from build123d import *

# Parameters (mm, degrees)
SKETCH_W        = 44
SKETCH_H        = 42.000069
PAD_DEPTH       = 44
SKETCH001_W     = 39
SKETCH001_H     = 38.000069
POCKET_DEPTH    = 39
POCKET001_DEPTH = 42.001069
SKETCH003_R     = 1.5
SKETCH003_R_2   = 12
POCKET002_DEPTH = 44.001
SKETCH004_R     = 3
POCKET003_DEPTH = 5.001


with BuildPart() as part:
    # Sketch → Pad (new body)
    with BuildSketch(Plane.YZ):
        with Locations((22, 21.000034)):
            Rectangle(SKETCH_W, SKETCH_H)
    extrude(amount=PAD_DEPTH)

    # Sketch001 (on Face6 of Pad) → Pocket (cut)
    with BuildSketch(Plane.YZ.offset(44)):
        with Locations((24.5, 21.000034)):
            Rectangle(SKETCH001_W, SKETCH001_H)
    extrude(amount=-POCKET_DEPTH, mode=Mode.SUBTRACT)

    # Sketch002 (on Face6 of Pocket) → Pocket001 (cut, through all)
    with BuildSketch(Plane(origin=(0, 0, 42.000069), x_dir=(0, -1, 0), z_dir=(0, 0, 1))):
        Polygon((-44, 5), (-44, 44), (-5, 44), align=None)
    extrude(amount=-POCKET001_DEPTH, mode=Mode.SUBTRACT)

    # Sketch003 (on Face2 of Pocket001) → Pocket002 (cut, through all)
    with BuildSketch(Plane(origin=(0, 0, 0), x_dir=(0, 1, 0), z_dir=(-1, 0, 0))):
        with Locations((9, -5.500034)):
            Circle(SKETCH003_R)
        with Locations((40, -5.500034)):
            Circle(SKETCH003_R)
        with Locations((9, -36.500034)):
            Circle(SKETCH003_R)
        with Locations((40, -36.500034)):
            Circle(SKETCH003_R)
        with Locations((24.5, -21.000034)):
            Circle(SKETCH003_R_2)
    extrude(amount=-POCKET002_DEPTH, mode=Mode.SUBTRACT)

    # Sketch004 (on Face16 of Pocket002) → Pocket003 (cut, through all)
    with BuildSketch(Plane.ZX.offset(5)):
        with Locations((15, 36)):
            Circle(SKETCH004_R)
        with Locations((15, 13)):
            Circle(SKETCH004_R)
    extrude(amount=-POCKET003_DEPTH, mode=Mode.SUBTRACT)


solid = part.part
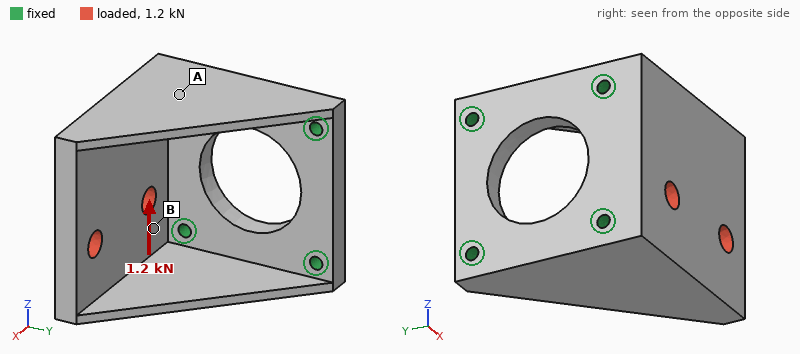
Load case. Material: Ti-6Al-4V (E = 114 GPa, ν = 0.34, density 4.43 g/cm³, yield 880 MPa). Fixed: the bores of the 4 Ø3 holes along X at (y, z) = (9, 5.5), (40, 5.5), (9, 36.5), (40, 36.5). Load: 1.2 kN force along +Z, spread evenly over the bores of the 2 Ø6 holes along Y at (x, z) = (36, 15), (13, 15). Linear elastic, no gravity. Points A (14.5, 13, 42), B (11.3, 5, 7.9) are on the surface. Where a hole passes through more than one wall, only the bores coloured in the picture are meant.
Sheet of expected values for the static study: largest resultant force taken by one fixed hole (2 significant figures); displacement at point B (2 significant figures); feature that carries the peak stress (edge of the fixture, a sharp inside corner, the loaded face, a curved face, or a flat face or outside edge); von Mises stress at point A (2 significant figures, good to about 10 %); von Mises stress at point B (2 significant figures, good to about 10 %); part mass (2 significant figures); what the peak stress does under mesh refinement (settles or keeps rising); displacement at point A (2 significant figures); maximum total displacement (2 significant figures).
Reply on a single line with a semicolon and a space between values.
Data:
1.1 kN; 5.0 µm; edge of the fixture; 8.3 MPa; 17 MPa; 79 g; keeps rising; 5.2 µm; 17 µm
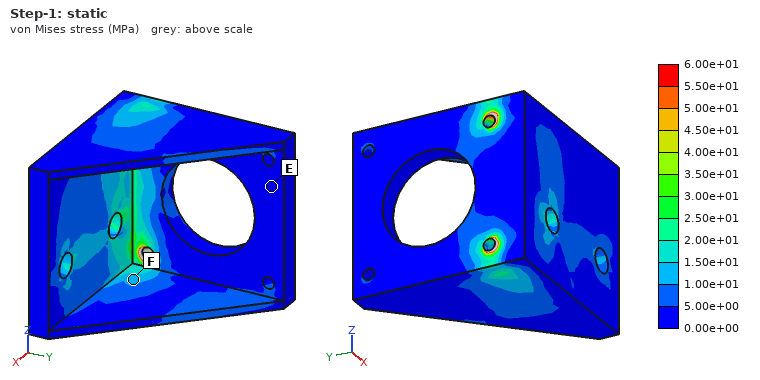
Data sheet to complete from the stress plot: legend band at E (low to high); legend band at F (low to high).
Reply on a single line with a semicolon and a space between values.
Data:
0.00e+00 to 5.00e+00 MPa; 1.00e+01 to 1.50e+01 MPa
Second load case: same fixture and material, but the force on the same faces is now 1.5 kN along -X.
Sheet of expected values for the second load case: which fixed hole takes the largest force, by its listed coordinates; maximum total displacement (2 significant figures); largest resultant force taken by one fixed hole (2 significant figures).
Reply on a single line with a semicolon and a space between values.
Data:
(9, 5.5); 13 µm; 1.1 kN
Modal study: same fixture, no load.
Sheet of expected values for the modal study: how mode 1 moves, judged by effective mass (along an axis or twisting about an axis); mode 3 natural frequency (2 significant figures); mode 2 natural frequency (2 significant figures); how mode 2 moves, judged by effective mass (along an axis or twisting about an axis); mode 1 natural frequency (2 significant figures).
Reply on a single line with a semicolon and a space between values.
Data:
along Y; 8100 Hz; 6900 Hz; along Z; 5700 Hz
